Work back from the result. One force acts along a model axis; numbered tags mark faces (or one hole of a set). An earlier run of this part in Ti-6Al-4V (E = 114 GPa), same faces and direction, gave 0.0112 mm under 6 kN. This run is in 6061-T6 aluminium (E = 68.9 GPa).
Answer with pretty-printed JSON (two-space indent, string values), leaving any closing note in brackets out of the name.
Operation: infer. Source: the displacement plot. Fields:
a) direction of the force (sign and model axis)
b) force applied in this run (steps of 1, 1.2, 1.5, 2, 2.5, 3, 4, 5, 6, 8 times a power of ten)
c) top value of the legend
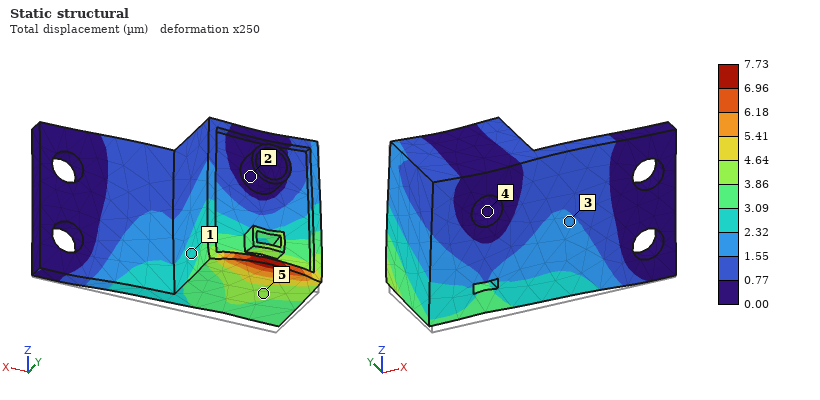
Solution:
{
  "direction of the force": "+Z",
  "force applied in this run": "2.5 kN",
  "top value of the legend": "7.73 µm"
}
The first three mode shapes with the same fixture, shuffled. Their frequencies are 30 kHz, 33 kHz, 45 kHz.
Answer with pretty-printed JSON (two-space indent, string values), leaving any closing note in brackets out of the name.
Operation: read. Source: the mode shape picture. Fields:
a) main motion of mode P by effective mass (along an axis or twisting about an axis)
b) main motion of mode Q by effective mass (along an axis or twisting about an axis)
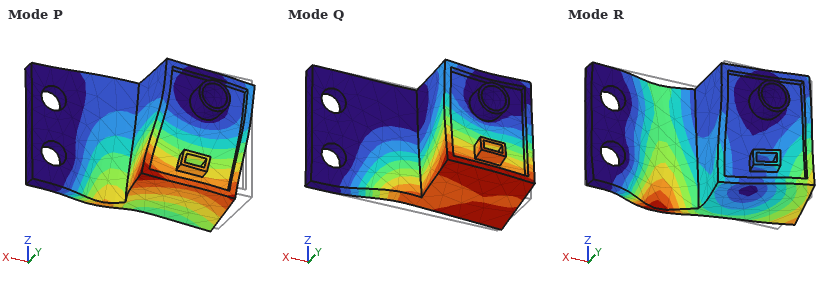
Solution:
{
  "main motion of mode P by effective mass": "along X",
  "main motion of mode Q by effective mass": "along Y"
}
